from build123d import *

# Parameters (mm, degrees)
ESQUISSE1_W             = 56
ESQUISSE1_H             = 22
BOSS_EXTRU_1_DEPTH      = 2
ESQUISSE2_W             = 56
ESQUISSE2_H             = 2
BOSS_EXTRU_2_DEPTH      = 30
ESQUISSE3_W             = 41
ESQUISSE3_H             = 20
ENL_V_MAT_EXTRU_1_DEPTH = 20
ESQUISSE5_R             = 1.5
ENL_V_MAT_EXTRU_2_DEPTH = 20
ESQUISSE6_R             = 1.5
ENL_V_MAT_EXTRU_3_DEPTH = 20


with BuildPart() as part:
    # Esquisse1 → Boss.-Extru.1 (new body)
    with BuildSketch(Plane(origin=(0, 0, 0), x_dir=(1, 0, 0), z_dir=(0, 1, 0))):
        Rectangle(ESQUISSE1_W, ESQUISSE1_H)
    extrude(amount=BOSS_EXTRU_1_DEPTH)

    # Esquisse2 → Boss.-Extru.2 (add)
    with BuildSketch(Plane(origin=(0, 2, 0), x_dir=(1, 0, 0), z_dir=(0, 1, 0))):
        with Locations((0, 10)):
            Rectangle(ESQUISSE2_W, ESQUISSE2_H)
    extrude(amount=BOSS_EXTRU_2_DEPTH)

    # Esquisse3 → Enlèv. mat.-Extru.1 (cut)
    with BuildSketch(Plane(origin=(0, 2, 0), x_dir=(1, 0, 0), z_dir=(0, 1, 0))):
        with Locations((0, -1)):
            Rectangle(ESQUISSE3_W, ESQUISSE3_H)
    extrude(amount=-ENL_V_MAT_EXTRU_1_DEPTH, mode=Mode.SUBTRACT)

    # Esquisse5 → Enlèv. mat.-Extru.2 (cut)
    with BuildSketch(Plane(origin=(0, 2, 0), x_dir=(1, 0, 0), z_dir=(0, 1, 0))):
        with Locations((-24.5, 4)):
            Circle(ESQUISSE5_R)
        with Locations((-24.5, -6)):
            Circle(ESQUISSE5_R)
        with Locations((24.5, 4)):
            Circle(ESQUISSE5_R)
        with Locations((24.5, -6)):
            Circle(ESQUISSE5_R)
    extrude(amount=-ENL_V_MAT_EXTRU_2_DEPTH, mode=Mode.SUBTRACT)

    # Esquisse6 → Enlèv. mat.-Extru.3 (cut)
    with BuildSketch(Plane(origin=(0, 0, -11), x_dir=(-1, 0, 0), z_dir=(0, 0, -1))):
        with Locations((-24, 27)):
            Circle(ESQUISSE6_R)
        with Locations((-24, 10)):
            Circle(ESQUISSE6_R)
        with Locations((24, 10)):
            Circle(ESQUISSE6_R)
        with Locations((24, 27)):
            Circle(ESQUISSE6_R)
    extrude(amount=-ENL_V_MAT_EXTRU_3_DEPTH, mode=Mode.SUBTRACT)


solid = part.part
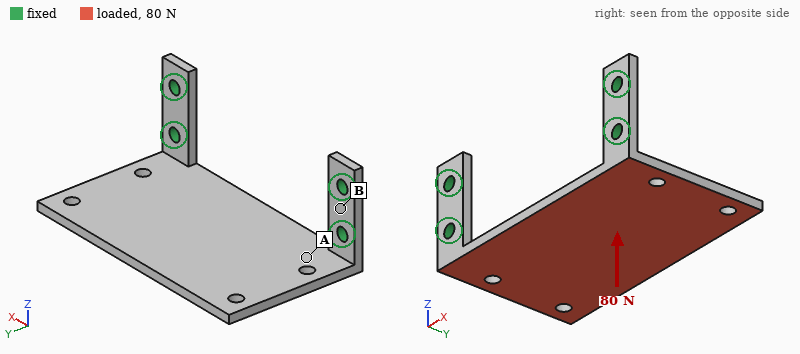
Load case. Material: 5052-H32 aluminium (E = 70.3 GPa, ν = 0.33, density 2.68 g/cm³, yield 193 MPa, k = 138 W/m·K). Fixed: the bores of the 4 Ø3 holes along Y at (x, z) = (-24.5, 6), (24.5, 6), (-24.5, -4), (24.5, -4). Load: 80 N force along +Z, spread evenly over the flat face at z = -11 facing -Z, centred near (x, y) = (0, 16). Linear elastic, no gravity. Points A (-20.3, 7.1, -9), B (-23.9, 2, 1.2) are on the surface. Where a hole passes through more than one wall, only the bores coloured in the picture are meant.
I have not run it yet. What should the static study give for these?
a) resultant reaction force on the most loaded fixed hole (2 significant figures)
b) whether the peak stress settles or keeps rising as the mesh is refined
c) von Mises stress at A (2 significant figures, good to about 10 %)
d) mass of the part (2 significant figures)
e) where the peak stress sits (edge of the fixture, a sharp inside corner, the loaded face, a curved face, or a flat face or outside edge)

39 N
keeps rising
37 MPa
11 g
edge of the fixture
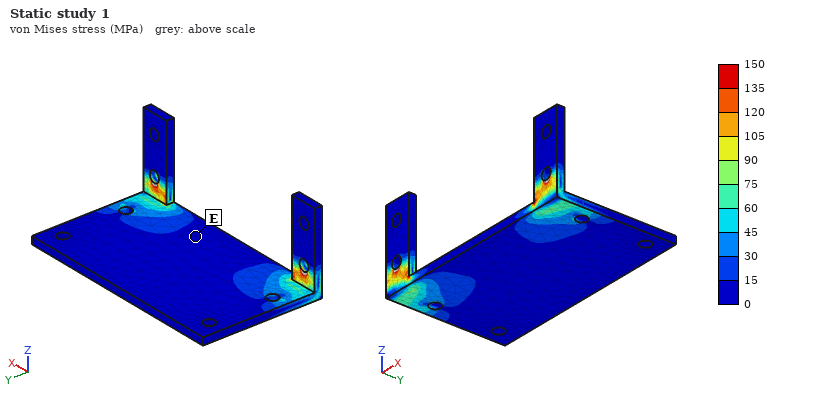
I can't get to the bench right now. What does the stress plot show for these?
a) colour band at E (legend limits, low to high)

0 to 15 MPa
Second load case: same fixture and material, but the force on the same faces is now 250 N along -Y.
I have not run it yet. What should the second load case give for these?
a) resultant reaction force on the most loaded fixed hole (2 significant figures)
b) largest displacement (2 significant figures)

130 N
0.26 mm
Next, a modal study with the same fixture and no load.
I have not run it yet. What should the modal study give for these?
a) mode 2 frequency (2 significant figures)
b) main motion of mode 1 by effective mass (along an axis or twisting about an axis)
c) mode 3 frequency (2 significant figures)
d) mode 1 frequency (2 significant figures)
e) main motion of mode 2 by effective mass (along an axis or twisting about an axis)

2300 Hz
along Z
4300 Hz
820 Hz
twisting about Y
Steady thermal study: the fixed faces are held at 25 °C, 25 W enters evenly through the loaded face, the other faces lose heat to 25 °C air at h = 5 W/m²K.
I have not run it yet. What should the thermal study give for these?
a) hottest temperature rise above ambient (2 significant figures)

77 K
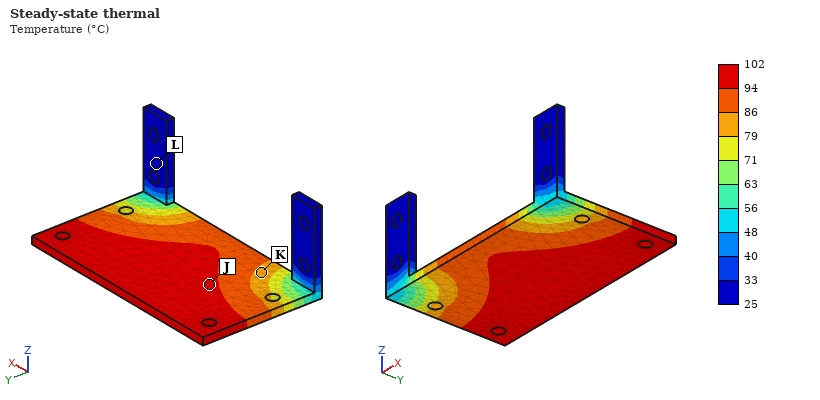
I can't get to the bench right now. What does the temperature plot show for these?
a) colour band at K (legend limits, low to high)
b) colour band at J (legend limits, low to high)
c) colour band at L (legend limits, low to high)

79 to 86 °C
94 to 102 °C
25 to 33 °C
